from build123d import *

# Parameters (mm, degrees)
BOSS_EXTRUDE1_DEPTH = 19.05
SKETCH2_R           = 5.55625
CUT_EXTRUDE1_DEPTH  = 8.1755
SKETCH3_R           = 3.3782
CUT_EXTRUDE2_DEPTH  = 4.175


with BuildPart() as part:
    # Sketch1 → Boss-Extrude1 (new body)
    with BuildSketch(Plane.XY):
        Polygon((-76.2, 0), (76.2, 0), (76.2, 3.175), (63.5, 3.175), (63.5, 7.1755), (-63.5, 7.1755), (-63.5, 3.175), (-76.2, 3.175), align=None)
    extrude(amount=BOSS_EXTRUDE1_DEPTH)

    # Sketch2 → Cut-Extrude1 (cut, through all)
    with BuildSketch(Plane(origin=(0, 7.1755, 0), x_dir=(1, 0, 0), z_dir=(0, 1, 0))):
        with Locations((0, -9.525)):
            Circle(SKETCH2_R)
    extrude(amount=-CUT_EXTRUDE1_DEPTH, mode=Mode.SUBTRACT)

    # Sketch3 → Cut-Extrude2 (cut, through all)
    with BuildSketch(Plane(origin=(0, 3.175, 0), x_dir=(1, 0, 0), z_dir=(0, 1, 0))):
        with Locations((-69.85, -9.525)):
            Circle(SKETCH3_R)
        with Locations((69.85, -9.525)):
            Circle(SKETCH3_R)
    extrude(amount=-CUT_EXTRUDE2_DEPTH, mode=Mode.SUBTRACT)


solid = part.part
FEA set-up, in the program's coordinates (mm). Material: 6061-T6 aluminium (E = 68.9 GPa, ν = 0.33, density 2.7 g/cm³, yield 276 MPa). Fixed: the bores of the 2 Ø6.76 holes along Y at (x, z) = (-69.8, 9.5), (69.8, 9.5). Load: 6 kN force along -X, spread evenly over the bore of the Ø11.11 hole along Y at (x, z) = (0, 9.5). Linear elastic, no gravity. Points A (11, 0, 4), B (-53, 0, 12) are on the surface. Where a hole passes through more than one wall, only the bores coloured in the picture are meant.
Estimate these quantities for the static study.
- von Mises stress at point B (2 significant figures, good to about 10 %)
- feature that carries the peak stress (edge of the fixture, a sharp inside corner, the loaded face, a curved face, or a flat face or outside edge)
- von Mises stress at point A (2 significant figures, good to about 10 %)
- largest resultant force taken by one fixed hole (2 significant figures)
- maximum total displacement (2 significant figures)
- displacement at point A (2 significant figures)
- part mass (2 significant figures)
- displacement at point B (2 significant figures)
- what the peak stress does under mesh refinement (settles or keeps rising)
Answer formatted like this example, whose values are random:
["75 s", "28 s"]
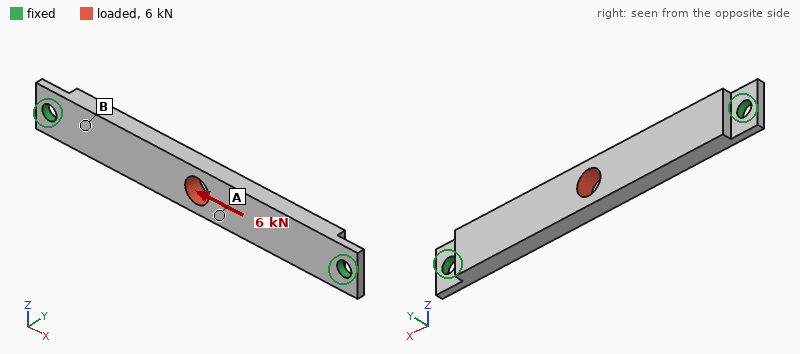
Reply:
["46 MPa", "edge of the fixture", "28 MPa", "3.0 kN", "36 µm", "33 µm", "49 g", "23 µm", "keeps rising"]
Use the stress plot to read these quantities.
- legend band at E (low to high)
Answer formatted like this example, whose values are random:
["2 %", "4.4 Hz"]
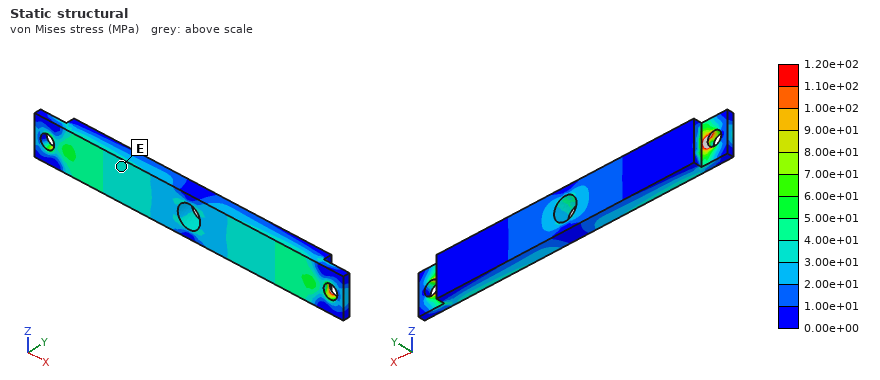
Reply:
["3.00e+01 to 4.00e+01 MPa"]
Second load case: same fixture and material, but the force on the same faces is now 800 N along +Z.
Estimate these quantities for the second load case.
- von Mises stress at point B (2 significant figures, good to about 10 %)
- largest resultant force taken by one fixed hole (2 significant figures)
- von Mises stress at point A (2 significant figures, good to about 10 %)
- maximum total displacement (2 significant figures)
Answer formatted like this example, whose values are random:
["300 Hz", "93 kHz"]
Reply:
["10 MPa", "400 N", "17 MPa", "83 µm"]
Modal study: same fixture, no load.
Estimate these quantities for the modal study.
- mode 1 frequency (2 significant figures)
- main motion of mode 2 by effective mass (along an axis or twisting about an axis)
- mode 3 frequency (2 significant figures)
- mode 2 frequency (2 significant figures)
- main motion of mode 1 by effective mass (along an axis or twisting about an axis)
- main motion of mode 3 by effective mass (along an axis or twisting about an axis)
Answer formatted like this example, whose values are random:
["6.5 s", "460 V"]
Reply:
["1300 Hz", "along Z", "4000 Hz", "3400 Hz", "along Y", "twisting about Z"]
